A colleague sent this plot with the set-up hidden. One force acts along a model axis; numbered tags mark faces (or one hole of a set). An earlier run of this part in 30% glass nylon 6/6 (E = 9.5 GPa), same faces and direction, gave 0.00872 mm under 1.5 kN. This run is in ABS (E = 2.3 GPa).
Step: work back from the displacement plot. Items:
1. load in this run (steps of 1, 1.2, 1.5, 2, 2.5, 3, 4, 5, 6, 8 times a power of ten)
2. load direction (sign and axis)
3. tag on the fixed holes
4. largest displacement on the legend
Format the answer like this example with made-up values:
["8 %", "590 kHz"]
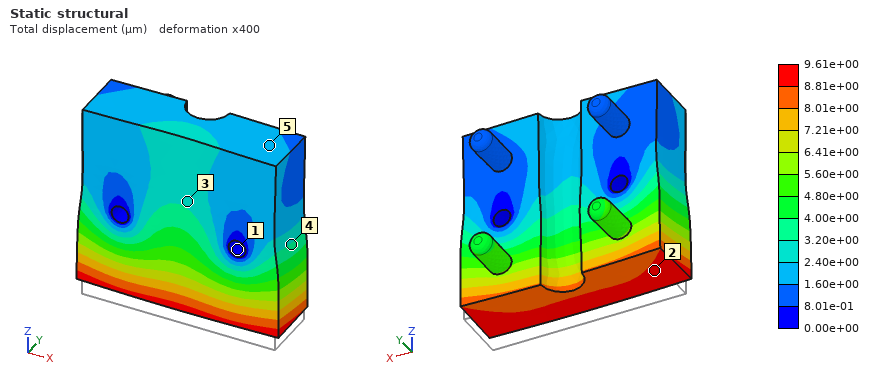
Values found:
["400 N", "+Z", "1", "9.61e+00 µm"]
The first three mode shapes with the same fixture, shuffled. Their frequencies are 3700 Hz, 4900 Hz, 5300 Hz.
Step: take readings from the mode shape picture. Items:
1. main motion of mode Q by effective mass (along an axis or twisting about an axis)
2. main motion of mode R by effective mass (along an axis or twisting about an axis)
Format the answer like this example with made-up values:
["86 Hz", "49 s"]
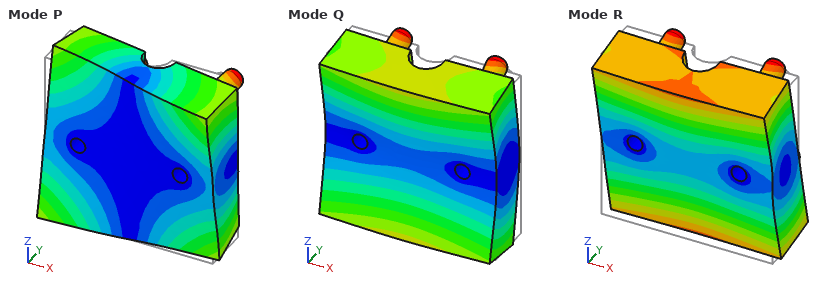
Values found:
["along Y", "twisting about X"]
